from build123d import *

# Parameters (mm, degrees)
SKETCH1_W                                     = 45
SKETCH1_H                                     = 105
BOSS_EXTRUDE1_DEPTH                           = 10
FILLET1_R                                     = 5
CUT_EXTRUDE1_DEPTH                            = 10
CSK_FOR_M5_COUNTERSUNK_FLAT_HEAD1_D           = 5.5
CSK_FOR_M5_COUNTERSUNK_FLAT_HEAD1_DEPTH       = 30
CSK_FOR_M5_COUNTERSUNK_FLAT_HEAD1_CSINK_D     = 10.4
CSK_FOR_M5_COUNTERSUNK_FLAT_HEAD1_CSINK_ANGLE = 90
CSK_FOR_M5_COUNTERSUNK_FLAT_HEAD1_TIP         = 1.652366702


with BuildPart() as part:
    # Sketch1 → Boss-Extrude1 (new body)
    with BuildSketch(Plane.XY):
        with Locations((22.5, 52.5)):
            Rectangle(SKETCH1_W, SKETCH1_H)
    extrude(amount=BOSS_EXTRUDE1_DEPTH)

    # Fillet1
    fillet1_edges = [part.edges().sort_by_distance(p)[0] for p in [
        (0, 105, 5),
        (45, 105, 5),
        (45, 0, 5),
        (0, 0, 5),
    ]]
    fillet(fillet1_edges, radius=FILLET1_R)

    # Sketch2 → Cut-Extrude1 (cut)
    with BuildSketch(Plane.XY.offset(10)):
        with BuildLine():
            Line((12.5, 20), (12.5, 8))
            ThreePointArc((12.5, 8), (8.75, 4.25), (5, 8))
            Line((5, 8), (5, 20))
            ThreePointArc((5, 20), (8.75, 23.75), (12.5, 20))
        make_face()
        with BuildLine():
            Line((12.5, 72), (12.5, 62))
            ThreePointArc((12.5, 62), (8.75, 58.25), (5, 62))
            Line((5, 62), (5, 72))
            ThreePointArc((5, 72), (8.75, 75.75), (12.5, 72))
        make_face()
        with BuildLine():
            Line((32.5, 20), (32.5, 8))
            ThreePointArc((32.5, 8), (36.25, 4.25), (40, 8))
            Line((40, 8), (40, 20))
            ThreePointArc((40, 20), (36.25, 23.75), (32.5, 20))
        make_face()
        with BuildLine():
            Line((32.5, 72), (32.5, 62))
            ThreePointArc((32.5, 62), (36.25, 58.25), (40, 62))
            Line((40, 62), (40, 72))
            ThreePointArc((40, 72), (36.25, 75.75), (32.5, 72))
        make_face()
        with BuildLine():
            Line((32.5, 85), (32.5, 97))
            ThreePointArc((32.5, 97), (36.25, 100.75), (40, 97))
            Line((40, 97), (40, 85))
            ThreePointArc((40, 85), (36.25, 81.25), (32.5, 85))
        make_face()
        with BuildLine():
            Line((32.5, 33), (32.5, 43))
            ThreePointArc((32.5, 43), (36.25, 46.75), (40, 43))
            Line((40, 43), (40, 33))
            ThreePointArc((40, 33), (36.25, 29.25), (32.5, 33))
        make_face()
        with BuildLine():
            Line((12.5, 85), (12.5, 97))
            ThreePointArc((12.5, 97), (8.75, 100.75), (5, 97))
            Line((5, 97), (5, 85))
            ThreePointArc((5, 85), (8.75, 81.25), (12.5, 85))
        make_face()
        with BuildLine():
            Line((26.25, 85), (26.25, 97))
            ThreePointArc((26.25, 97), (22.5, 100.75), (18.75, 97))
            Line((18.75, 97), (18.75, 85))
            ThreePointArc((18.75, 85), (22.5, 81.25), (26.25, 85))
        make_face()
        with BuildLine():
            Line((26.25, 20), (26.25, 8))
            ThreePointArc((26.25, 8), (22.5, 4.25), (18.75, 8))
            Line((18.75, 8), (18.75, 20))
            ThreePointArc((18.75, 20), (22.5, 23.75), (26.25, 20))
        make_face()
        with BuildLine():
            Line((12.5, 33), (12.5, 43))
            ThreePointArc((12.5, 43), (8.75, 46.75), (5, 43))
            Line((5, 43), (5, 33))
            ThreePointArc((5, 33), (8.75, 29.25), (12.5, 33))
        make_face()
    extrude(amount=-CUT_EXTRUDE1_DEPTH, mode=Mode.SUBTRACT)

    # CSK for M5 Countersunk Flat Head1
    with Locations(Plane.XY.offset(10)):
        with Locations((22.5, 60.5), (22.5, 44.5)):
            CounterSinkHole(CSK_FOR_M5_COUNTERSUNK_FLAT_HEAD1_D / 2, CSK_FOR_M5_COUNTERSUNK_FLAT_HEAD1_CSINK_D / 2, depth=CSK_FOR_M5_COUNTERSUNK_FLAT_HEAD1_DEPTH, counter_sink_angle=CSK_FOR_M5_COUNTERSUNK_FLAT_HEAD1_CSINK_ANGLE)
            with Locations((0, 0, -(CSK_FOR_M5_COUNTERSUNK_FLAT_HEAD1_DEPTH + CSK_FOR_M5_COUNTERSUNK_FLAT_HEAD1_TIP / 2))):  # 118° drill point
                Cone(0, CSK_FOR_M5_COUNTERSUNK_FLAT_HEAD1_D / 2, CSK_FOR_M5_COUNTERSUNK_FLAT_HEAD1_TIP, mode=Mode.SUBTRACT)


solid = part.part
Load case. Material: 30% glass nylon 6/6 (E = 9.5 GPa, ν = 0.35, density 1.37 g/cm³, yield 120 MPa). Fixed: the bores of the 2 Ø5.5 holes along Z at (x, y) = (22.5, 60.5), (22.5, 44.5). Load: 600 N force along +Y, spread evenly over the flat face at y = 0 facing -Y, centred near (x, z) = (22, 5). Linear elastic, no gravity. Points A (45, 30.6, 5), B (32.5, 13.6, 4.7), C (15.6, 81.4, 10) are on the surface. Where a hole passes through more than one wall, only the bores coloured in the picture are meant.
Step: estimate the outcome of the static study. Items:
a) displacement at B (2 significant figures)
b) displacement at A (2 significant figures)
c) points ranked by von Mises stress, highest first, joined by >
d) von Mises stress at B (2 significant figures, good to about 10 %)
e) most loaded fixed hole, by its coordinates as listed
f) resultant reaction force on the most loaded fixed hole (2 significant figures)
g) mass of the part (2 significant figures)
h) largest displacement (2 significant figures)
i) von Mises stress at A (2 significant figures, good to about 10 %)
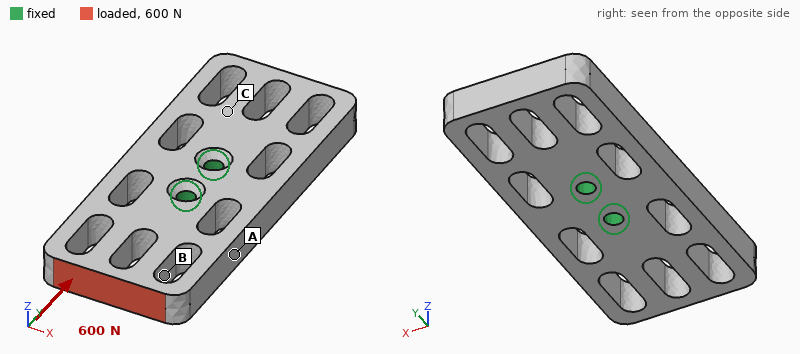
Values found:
11 µm
6.6 µm
B > A > C
3.5 MPa
(22.5, 44.5)
440 N
46 g
18 µm
1.7 MPa
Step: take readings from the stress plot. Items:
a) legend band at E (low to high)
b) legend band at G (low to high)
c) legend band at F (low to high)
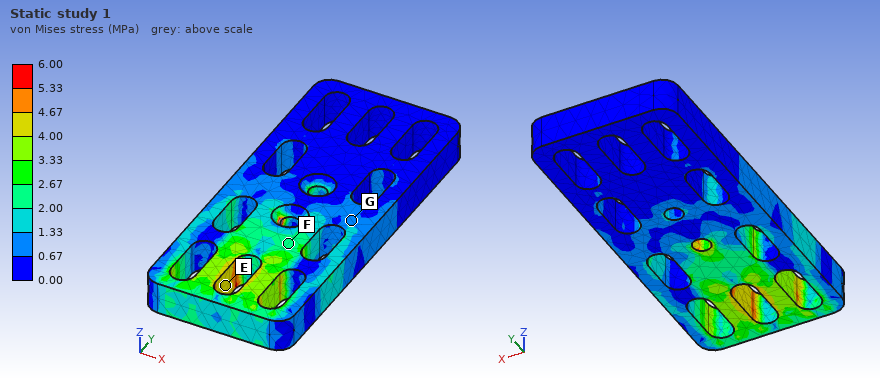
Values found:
4.00 to 4.67 MPa
0.67 to 1.33 MPa
2.00 to 2.67 MPa
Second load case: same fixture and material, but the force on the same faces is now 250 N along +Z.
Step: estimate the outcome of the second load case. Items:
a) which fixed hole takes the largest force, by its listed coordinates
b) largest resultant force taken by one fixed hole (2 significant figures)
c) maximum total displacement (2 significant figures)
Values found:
(22.5, 44.5)
540 N
0.40 mm
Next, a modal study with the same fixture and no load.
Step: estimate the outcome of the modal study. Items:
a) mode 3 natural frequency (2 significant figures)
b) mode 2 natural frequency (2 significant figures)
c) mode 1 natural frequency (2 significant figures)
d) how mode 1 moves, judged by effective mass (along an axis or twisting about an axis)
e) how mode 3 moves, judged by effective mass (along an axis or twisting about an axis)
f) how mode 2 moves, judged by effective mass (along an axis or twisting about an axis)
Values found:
2700 Hz
1900 Hz
1800 Hz
twisting about X
twisting about Z
along Z
